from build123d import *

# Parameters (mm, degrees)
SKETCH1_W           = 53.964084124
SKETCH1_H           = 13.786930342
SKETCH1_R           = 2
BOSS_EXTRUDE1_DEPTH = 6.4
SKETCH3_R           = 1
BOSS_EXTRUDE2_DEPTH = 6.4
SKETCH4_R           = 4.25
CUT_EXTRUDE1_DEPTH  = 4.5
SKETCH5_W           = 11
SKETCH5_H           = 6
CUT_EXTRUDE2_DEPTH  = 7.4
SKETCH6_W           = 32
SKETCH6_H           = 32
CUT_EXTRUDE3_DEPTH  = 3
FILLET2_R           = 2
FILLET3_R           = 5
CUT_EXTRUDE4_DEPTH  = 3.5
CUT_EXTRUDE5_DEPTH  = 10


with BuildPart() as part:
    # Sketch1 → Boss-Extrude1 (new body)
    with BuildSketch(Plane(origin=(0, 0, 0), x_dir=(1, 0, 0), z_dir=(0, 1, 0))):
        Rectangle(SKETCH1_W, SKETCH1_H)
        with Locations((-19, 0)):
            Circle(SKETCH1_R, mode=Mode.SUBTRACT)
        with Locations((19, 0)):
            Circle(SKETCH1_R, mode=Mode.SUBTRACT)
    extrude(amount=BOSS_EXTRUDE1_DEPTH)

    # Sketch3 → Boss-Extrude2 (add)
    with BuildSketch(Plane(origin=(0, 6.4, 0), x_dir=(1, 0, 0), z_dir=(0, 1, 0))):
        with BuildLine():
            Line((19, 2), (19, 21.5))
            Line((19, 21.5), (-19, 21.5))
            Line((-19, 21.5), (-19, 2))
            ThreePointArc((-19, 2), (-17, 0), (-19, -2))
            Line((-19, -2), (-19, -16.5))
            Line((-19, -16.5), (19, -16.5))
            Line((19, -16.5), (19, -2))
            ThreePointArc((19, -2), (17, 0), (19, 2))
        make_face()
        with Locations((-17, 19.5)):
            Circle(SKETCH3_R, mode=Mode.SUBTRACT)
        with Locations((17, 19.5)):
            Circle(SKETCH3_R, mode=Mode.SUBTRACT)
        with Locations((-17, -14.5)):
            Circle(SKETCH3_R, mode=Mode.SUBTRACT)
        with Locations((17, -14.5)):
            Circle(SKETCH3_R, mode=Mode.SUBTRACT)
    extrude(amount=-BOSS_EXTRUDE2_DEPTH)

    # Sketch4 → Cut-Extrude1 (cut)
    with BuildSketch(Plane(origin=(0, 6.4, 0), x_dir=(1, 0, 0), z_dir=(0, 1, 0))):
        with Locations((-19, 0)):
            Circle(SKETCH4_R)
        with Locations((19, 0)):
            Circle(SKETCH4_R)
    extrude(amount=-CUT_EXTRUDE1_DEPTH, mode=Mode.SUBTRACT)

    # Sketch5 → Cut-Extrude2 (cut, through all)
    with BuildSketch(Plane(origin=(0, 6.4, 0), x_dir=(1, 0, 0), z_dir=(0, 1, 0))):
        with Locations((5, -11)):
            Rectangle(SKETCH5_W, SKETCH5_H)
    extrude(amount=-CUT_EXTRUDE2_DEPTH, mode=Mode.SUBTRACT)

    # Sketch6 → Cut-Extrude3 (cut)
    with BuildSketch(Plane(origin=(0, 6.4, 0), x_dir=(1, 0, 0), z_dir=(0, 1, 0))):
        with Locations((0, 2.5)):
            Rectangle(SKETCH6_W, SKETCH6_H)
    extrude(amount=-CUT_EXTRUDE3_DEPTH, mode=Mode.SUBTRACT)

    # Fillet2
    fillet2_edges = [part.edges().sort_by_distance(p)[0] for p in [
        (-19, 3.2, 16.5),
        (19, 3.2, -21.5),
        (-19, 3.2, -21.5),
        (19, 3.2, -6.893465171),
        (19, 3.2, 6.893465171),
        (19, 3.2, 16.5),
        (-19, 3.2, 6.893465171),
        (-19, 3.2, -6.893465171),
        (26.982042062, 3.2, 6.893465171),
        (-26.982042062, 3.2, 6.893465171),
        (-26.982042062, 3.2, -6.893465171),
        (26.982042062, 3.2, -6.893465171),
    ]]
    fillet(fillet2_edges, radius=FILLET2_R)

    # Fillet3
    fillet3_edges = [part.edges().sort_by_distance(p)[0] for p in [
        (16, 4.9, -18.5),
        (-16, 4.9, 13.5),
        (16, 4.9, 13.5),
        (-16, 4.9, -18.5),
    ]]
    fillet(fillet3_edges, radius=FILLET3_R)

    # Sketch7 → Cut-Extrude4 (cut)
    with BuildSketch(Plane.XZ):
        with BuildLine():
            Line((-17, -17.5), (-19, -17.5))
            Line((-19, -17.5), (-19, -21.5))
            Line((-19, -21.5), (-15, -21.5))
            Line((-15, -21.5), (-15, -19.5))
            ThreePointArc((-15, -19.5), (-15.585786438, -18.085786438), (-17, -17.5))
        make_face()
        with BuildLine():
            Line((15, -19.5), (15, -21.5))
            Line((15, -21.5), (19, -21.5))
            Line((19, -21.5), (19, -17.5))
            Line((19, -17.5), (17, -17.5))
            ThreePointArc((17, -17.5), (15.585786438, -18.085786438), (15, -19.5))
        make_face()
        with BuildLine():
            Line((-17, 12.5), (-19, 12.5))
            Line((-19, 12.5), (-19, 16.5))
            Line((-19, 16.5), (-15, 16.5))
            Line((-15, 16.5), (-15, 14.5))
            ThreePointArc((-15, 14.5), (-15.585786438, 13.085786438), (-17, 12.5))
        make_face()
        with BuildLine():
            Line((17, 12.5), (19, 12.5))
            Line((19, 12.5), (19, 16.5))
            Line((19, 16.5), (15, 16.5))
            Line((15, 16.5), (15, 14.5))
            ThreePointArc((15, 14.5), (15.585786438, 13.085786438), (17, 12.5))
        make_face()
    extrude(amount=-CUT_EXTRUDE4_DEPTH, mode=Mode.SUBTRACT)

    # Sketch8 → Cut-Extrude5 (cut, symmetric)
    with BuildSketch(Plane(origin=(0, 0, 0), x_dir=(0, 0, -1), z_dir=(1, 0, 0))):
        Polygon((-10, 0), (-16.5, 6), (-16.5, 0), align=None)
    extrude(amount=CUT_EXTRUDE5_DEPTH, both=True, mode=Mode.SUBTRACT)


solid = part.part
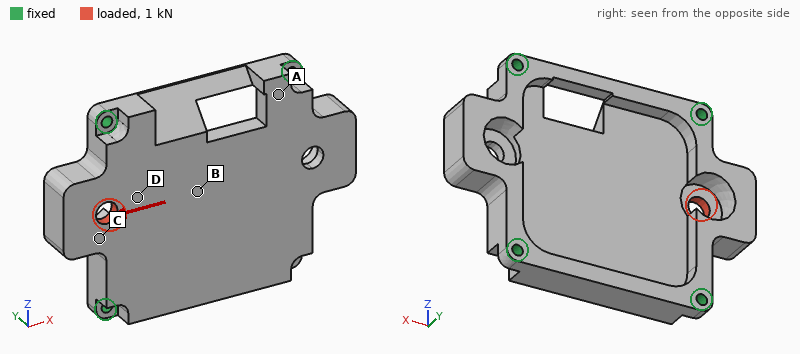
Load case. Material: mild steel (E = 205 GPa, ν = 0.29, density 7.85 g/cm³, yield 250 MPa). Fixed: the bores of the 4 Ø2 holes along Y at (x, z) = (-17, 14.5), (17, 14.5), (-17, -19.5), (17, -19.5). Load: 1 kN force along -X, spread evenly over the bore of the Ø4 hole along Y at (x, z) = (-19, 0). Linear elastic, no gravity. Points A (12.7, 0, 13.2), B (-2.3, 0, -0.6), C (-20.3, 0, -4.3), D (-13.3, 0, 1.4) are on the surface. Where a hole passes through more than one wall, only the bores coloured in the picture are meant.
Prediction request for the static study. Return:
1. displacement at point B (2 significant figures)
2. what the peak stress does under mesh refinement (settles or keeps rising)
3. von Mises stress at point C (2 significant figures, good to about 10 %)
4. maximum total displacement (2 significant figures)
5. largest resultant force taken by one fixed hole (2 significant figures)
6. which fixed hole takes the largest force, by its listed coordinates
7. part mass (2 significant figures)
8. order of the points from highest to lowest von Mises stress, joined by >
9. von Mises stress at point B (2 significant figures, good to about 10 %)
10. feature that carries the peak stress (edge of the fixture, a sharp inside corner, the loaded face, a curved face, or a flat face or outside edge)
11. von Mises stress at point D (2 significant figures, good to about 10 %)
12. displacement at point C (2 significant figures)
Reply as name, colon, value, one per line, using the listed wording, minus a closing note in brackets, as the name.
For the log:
displacement at point B: 2.4 µm
what the peak stress does under mesh refinement: keeps rising
von Mises stress at point C: 23 MPa
maximum total displacement: 6.5 µm
largest resultant force taken by one fixed hole: 340 N
which fixed hole takes the largest force, by its listed coordinates: (17, -19.5)
part mass: 49 g
order of the points from highest to lowest von Mises stress, joined by >: D > C > B > A
von Mises stress at point B: 16 MPa
feature that carries the peak stress: edge of the fixture
von Mises stress at point D: 35 MPa
displacement at point C: 3.8 µm
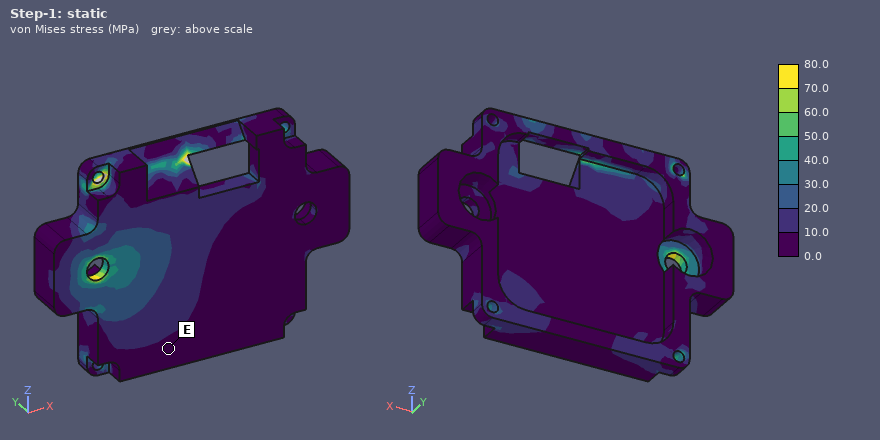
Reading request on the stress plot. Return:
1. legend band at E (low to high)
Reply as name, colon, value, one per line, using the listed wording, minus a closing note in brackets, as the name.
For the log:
legend band at E: 0.0 to 10.0 MPa
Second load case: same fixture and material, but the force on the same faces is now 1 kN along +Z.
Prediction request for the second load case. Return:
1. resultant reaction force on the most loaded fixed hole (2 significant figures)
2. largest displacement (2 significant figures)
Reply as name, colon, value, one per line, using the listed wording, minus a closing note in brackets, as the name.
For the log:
resultant reaction force on the most loaded fixed hole: 480 N
largest displacement: 3.5 µm
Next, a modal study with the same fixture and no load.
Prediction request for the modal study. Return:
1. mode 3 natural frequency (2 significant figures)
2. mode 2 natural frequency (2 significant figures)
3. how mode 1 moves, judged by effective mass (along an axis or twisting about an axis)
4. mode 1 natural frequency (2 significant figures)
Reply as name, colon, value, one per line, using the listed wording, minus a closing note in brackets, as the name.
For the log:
mode 3 natural frequency: 11 kHz
mode 2 natural frequency: 11 kHz
how mode 1 moves, judged by effective mass: along Y
mode 1 natural frequency: 11 kHz
